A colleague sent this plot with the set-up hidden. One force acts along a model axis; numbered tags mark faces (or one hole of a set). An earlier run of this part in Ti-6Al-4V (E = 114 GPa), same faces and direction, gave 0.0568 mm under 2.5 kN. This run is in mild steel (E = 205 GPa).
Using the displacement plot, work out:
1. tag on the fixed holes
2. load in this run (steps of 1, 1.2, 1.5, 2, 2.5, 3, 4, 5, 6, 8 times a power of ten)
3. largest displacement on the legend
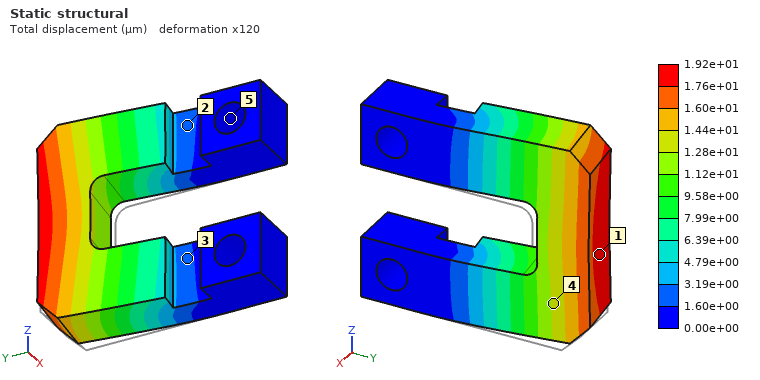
5
1.5 kN
1.92e+01 µm
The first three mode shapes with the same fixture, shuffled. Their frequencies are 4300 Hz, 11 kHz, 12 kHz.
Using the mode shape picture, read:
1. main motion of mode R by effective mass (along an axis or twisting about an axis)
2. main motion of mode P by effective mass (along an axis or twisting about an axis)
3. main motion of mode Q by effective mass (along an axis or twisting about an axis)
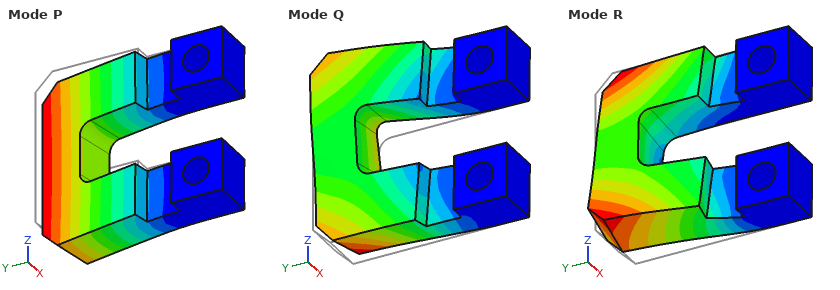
along Z
along X
along Z
